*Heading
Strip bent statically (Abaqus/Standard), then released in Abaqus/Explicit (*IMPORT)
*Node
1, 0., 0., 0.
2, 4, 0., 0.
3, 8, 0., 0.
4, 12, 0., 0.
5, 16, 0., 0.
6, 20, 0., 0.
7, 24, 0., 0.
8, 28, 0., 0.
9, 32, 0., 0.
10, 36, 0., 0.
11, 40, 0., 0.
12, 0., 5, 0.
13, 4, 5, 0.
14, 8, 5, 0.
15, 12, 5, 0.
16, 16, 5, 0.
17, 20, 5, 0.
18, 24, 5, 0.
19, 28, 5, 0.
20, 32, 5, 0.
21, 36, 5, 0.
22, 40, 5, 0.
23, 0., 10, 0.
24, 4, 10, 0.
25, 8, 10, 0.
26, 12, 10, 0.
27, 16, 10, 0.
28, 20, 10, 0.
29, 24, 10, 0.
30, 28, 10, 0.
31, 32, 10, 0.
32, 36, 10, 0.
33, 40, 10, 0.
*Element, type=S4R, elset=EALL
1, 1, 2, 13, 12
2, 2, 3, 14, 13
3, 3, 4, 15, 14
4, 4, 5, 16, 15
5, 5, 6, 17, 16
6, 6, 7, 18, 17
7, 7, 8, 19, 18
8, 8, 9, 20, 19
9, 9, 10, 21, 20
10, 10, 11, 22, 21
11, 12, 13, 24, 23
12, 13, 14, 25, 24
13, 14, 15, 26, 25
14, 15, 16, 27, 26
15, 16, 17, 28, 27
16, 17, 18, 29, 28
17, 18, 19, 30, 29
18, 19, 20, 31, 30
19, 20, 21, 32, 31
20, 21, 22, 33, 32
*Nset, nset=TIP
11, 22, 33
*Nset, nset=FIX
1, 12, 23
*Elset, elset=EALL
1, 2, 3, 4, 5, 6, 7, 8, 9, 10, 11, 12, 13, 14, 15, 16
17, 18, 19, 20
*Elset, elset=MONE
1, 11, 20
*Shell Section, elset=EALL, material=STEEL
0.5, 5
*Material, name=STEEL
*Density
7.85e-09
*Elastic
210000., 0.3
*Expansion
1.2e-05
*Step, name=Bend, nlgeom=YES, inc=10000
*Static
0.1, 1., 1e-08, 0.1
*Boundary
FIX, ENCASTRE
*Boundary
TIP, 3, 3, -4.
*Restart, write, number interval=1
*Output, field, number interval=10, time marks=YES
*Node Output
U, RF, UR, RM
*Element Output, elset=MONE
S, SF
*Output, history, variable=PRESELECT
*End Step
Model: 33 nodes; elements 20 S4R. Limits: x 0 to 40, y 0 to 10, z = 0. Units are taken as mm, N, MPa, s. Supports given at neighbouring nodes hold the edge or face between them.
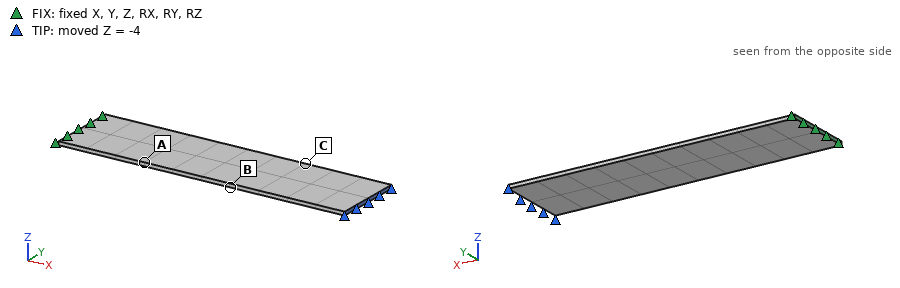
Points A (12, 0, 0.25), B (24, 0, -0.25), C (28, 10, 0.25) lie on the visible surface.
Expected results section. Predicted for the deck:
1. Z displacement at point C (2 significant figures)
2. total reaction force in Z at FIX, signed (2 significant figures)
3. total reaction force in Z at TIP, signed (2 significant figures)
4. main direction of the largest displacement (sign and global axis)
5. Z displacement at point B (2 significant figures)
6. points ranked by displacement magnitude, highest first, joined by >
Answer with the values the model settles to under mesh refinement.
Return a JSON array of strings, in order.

["-2.2 mm", "4.3 N", "-4.3 N", "-Z", "-1.7 mm", "C > B > A"]
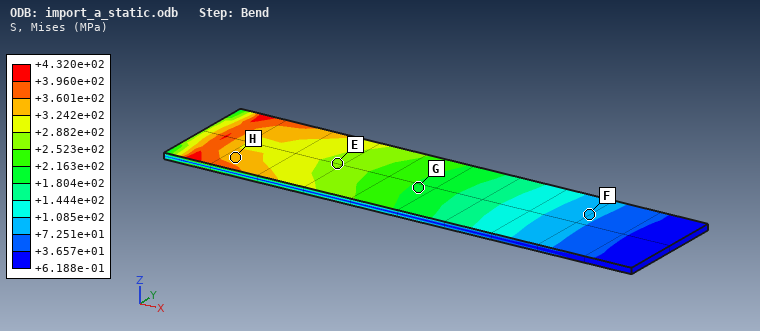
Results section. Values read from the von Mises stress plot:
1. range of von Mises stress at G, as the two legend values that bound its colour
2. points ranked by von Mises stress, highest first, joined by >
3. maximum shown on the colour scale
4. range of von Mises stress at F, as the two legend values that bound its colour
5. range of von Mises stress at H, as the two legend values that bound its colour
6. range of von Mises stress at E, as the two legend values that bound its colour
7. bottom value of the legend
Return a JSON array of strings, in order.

["+1.804e+02 to +2.163e+02 MPa", "H > E > G > F", "+4.320e+02 MPa", "+7.251e+01 to +1.085e+02 MPa", "+3.242e+02 to +3.601e+02 MPa", "+2.523e+02 to +2.882e+02 MPa", "+6.188e-01 MPa"]
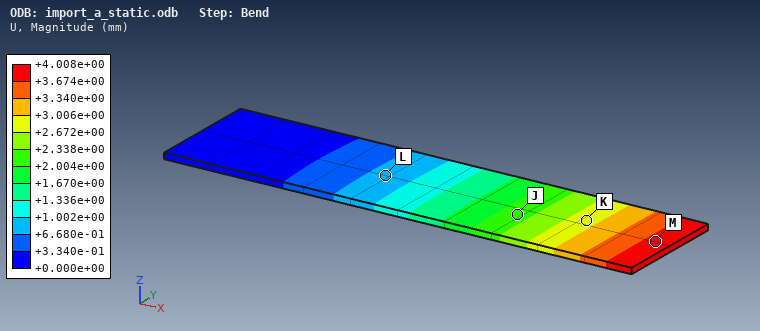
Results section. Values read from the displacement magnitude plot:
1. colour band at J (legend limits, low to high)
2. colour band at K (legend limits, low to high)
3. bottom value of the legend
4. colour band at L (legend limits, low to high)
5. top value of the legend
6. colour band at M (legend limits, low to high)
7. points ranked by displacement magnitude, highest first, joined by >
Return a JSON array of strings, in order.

["+2.004e+00 to +2.338e+00 mm", "+2.672e+00 to +3.006e+00 mm", "+0.000e+00 mm", "+6.680e-01 to +1.002e+00 mm", "+4.008e+00 mm", "+3.674e+00 to +4.008e+00 mm", "M > K > J > L"]
